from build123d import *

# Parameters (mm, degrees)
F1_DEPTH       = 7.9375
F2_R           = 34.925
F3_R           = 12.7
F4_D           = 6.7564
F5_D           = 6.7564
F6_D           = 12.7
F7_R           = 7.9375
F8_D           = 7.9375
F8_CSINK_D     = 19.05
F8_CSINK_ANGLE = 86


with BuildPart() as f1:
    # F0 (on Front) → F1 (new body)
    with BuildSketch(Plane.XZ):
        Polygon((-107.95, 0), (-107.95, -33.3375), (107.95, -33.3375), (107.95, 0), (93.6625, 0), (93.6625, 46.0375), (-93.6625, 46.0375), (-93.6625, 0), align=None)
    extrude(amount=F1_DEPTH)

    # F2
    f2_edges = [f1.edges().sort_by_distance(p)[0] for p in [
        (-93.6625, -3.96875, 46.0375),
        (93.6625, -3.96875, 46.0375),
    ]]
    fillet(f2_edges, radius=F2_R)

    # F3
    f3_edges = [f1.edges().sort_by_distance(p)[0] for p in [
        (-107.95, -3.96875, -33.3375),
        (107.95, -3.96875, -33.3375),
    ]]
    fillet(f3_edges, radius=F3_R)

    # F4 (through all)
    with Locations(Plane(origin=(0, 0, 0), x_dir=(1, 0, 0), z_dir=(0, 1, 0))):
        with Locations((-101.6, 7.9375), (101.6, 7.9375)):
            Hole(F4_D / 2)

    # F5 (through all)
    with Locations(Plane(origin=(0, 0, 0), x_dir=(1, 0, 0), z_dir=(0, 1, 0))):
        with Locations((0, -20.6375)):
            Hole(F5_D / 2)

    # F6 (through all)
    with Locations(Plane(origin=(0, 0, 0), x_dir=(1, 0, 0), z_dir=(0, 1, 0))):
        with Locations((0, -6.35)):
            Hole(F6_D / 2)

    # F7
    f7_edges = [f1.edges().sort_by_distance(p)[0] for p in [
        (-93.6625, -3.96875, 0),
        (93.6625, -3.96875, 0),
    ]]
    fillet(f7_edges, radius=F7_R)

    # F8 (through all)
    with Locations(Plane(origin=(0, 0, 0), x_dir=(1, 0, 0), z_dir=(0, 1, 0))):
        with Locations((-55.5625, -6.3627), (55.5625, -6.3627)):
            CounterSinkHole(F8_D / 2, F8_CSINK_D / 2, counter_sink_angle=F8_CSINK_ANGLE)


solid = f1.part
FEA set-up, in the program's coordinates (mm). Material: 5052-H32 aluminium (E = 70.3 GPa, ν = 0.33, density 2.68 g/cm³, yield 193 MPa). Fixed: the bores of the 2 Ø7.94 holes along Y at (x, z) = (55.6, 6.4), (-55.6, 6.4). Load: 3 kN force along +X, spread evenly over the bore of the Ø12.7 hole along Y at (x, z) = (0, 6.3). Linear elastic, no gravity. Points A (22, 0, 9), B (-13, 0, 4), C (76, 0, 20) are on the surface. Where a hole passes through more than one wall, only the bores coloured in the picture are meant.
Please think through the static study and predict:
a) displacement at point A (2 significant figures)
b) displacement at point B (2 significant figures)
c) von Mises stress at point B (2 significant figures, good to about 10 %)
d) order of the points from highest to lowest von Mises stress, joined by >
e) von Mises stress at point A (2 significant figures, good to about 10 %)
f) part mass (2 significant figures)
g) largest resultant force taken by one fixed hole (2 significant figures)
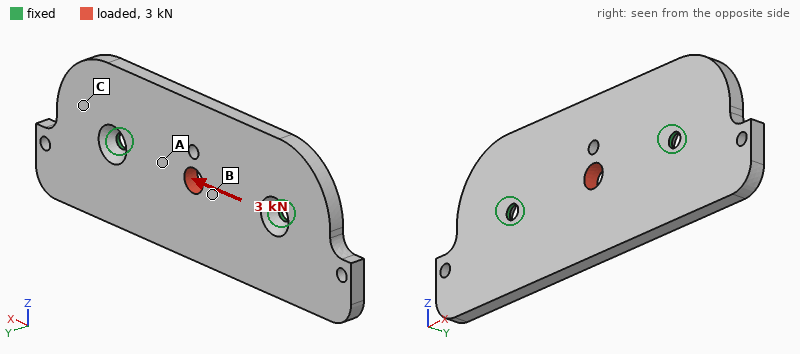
4.9 µm
5.3 µm
7.7 MPa
B > A > C
5.4 MPa
310 g
1.5 kN
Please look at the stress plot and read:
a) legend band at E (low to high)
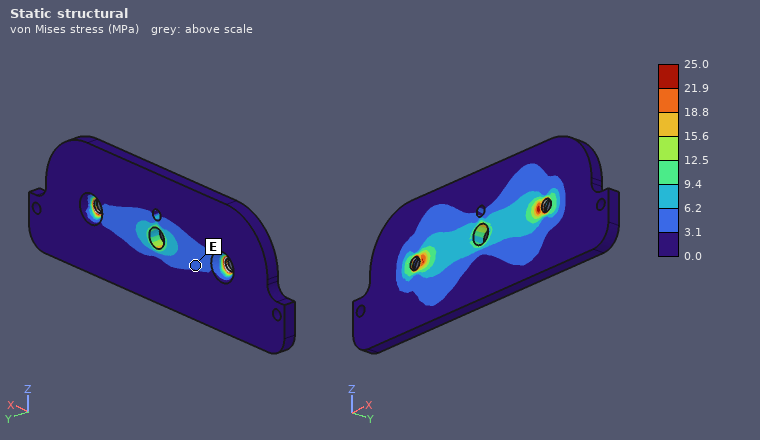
3.1 to 6.2 MPa
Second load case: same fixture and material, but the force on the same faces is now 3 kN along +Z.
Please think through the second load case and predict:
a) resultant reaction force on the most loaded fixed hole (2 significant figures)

1.5 kN
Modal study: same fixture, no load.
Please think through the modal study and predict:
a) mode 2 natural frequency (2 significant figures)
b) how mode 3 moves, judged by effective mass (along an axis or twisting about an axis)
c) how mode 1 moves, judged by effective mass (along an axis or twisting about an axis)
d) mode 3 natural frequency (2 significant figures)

1600 Hz
twisting about Z
twisting about X
1700 Hz
